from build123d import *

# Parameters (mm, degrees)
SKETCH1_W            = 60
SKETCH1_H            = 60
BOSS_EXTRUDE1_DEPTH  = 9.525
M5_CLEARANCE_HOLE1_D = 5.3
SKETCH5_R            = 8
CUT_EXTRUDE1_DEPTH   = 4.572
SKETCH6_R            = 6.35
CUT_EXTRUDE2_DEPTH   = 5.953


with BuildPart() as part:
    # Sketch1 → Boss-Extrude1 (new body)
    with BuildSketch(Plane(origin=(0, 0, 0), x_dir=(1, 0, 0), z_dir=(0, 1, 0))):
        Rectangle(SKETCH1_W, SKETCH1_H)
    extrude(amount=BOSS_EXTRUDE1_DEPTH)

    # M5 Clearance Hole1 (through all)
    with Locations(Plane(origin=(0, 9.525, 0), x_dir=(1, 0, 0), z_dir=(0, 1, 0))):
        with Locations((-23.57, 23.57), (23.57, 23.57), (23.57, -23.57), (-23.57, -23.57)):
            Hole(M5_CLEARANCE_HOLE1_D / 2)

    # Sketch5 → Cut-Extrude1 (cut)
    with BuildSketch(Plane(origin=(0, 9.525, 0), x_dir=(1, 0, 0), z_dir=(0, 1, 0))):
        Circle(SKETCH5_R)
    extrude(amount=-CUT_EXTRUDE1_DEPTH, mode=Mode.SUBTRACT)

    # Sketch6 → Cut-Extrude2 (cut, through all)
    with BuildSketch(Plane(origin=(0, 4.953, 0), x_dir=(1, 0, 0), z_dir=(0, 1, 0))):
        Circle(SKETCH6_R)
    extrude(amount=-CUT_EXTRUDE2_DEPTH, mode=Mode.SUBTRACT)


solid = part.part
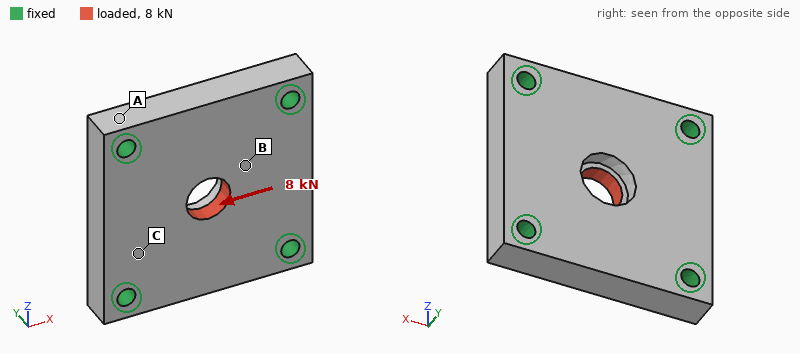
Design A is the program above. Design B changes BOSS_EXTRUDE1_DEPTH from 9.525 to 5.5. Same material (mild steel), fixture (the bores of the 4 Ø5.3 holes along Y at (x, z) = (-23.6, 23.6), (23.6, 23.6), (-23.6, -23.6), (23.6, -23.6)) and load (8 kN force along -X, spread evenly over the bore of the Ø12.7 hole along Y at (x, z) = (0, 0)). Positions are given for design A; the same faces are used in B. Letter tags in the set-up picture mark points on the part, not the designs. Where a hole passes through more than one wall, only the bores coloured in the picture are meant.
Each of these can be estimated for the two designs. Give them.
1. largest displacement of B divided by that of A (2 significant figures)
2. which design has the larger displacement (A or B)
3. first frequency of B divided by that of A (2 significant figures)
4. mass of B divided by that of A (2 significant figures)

1.3
B
0.67
0.58
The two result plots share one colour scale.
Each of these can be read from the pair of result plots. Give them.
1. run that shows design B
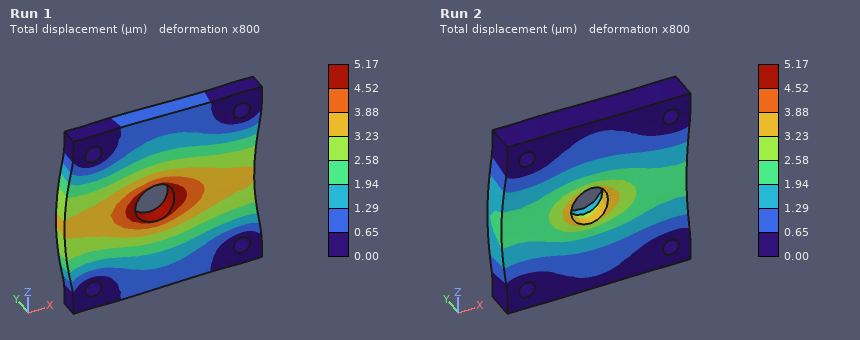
Run 1
